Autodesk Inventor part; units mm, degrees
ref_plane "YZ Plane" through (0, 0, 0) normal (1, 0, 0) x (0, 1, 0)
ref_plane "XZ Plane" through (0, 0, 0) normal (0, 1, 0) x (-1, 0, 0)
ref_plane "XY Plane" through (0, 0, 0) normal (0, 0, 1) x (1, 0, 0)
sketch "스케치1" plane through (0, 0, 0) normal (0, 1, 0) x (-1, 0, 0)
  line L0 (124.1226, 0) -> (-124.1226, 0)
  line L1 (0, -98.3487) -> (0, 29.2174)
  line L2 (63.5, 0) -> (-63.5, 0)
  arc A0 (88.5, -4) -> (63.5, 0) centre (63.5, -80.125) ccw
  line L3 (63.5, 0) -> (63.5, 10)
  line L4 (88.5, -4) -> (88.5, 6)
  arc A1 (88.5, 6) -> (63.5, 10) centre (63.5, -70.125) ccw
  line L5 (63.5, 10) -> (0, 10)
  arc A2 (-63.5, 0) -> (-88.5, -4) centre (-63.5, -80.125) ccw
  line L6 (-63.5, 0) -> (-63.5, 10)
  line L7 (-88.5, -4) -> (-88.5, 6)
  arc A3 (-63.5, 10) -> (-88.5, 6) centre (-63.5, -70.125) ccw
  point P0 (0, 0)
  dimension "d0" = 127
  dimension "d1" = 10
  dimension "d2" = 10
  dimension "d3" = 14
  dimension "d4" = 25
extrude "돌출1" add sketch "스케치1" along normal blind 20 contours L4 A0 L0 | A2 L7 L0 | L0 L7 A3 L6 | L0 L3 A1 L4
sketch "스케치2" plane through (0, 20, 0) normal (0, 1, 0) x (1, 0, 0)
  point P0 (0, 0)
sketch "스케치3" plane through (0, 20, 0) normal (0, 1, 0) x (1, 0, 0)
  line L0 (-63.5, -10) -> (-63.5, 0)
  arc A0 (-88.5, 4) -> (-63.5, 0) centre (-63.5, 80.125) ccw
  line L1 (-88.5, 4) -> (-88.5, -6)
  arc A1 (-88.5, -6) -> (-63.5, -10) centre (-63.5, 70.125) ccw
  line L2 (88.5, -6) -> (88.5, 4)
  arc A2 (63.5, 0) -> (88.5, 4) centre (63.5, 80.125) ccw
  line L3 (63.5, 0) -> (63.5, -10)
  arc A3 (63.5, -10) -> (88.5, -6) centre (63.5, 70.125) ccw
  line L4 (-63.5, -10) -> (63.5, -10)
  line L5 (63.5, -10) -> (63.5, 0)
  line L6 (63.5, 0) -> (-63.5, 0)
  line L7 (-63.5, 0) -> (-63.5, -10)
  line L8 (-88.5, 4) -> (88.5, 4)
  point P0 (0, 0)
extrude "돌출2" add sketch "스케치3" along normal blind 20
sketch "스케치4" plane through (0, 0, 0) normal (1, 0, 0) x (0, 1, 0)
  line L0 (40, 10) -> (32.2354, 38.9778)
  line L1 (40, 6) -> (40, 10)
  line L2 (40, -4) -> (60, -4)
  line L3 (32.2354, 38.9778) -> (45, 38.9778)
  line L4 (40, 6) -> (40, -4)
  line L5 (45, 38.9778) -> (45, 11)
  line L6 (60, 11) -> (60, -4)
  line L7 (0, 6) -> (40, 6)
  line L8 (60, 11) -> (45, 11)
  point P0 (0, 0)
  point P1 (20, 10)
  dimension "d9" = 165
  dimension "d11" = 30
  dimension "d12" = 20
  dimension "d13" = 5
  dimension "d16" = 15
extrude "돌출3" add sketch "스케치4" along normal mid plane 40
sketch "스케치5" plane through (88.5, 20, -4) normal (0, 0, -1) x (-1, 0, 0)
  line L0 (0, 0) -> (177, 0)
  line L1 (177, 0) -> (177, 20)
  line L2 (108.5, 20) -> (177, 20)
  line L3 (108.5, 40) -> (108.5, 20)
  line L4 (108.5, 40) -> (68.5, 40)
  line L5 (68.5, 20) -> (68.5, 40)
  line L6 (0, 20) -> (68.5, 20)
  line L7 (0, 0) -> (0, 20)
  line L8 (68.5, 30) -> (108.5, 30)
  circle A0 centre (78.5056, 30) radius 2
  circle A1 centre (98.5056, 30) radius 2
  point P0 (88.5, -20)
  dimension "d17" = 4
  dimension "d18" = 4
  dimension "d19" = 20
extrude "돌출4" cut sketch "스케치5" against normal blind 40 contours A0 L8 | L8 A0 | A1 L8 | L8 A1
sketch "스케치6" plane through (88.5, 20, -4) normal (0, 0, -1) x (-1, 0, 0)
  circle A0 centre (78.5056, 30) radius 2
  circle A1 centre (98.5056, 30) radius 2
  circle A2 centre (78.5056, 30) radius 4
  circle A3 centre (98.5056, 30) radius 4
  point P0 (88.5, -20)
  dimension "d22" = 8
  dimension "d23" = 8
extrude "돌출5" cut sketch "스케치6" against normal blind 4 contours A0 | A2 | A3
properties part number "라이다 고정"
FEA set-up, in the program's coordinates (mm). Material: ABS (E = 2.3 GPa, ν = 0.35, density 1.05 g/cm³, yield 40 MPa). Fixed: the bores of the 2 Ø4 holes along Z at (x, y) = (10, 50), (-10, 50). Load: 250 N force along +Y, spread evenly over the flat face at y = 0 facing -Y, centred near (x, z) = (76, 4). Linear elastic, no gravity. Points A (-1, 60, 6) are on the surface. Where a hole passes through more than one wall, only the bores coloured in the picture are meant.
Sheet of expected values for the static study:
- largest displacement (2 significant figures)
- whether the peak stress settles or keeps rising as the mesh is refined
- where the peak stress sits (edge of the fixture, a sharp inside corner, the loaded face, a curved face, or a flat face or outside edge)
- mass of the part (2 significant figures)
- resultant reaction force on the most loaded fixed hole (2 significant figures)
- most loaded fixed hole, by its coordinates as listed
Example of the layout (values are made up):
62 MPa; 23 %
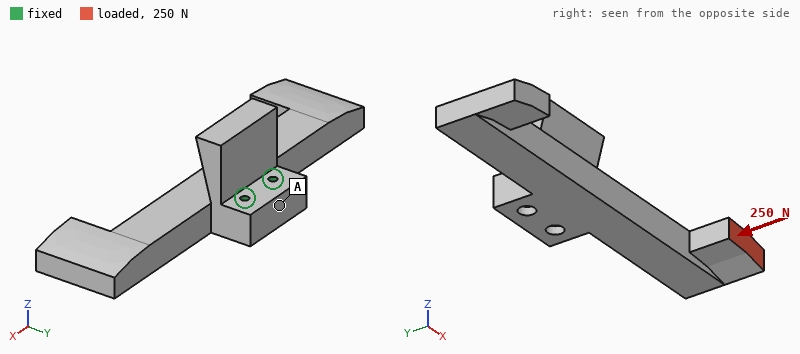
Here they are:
2.0 mm; keeps rising; edge of the fixture; 84 g; 1.0 kN; (10, 50)
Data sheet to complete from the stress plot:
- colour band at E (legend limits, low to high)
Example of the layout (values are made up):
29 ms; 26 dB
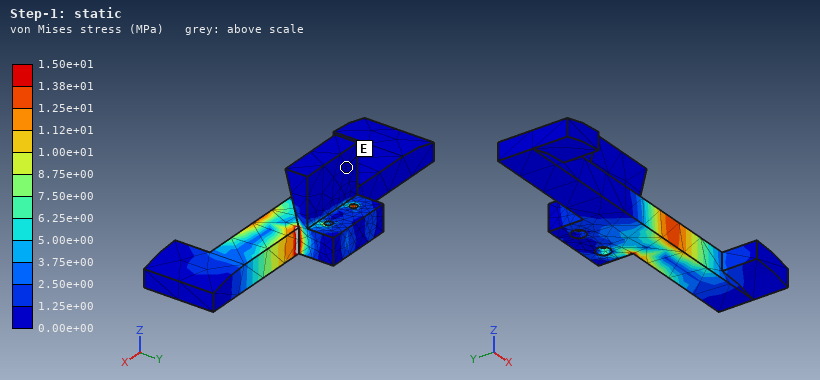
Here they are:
0.00e+00 to 1.25e+00 MPa
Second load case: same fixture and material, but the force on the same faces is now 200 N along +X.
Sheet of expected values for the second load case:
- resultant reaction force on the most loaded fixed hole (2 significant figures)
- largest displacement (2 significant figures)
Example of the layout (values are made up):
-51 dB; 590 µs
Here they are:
470 N; 1.2 mm
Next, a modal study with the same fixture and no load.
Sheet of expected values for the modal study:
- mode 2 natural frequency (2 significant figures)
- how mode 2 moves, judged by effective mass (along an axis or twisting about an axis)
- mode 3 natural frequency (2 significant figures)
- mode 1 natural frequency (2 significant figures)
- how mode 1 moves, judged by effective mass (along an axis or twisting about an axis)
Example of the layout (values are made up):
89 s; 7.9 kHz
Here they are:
390 Hz; along Z; 500 Hz; 340 Hz; twisting about Y
